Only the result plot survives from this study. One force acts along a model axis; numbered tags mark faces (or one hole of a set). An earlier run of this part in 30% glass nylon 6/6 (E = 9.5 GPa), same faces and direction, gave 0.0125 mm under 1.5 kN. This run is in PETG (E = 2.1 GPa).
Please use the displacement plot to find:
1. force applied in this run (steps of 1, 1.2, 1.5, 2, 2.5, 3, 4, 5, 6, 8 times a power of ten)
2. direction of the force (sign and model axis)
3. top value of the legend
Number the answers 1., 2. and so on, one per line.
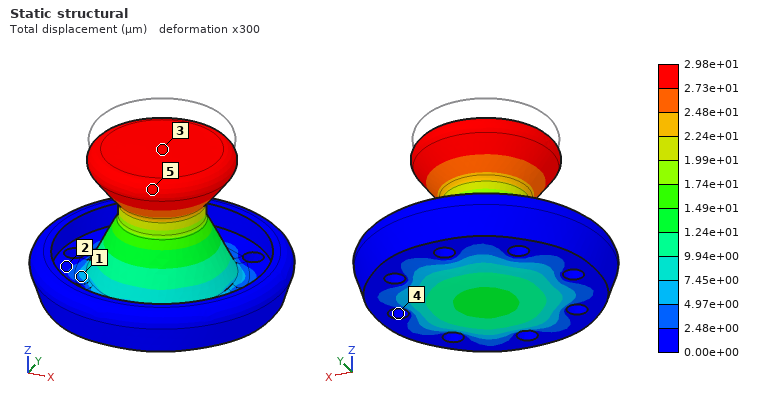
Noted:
1. 800 N
2. -Z
3. 2.98e+01 µm
